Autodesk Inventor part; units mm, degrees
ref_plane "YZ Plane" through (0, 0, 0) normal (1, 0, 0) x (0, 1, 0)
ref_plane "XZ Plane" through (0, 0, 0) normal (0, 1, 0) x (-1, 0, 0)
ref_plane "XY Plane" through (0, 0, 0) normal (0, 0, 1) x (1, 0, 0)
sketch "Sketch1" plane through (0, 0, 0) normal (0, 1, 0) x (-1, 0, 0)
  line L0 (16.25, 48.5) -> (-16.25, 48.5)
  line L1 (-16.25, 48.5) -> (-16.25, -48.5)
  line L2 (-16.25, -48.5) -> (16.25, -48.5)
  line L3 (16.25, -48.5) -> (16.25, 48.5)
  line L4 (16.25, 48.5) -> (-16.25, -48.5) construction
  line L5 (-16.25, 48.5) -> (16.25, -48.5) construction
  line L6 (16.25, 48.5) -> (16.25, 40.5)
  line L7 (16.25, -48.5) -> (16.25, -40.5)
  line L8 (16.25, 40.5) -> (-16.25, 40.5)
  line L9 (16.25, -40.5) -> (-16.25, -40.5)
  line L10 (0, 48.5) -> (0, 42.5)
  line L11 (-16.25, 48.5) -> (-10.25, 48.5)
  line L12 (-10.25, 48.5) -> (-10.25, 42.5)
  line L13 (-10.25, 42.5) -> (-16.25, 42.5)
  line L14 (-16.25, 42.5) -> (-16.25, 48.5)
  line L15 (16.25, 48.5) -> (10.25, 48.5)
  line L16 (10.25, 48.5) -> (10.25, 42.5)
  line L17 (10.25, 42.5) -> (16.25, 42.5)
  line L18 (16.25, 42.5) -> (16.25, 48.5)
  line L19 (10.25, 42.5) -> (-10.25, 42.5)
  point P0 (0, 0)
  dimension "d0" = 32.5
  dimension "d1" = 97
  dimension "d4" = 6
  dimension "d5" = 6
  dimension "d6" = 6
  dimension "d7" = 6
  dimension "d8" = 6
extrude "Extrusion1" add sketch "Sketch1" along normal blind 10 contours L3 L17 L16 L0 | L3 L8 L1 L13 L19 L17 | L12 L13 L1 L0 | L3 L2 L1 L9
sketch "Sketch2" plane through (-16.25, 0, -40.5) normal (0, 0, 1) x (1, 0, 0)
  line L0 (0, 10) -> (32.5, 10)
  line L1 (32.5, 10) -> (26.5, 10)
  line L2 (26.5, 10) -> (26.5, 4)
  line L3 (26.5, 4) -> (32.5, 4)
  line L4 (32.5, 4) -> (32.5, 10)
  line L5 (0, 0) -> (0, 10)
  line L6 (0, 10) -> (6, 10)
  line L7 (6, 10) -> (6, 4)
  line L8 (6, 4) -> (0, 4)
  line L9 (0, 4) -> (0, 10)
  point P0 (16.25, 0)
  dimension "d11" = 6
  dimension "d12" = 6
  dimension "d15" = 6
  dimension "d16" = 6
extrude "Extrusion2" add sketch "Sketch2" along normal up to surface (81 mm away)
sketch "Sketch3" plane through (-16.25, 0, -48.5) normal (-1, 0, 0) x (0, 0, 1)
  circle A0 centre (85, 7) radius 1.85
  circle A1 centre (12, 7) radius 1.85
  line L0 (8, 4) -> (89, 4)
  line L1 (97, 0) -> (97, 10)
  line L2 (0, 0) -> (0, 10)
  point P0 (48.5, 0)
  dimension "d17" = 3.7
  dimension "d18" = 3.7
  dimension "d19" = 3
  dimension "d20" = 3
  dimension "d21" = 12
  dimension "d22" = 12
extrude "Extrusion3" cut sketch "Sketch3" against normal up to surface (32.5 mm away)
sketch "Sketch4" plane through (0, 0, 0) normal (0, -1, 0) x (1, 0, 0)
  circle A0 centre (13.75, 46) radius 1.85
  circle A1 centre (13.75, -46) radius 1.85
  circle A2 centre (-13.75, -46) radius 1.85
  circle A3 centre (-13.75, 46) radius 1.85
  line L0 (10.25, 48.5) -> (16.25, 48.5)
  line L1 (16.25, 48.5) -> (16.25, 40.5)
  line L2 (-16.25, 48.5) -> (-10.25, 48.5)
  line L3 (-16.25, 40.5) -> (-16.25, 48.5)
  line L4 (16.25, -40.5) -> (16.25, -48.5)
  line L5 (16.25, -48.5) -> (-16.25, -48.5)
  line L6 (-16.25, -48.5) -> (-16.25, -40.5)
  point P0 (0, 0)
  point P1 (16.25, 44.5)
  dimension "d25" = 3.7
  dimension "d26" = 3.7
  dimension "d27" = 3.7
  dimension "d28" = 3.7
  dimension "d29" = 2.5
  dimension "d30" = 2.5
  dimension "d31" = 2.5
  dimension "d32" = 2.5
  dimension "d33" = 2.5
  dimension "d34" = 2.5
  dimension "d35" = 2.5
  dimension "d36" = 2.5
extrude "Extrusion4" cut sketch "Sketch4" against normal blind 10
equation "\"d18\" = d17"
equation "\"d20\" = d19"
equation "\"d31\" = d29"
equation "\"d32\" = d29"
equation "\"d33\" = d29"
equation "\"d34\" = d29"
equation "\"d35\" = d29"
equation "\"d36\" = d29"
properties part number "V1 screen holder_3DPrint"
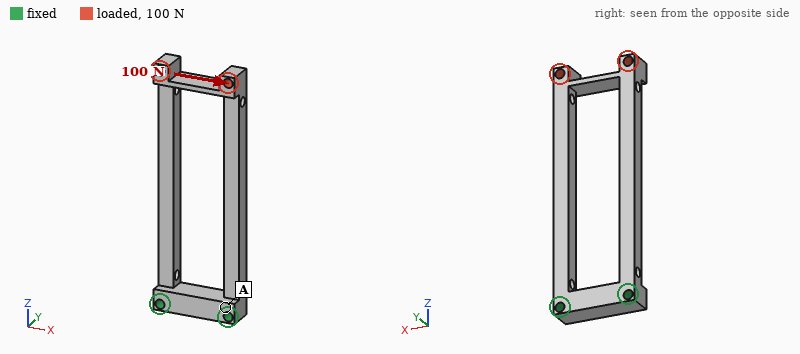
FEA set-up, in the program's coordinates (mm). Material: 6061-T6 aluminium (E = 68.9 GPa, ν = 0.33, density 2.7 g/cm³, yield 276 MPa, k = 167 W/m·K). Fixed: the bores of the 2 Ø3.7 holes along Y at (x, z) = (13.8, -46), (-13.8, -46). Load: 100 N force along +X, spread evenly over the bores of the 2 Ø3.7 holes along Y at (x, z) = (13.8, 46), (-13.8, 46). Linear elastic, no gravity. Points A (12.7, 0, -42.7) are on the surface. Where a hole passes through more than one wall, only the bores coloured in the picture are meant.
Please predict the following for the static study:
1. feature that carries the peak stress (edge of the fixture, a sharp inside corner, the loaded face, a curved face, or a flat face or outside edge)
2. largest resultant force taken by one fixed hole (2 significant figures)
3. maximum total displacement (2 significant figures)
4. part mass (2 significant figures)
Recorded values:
a curved face
240 N
0.93 mm
25 g
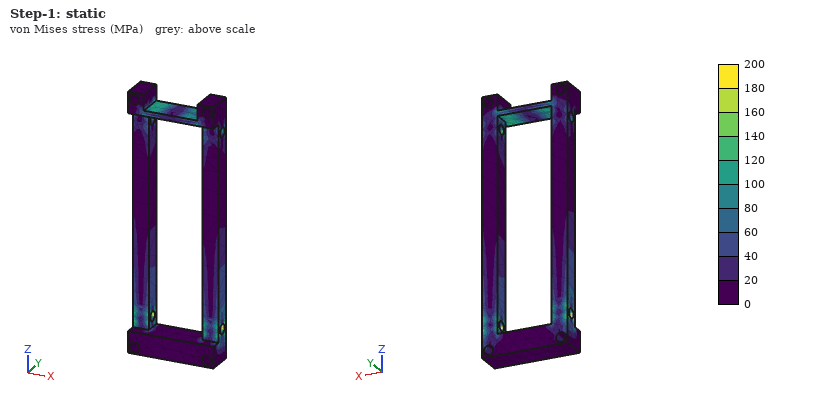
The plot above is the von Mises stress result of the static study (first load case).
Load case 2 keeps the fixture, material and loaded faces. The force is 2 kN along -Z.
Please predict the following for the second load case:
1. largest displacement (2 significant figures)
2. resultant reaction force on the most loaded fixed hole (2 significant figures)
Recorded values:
1.1 mm
1.0 kN
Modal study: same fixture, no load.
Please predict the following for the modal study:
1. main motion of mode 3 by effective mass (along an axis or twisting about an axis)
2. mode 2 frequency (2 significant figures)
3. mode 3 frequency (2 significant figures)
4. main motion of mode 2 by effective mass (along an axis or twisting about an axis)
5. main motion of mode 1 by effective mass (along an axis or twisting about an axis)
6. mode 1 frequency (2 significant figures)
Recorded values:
twisting about Z
630 Hz
1500 Hz
along X
along Y
520 Hz
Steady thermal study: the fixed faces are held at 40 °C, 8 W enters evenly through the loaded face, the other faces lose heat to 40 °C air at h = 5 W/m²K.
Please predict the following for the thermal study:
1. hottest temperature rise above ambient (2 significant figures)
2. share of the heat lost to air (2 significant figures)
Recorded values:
61 K
11 %
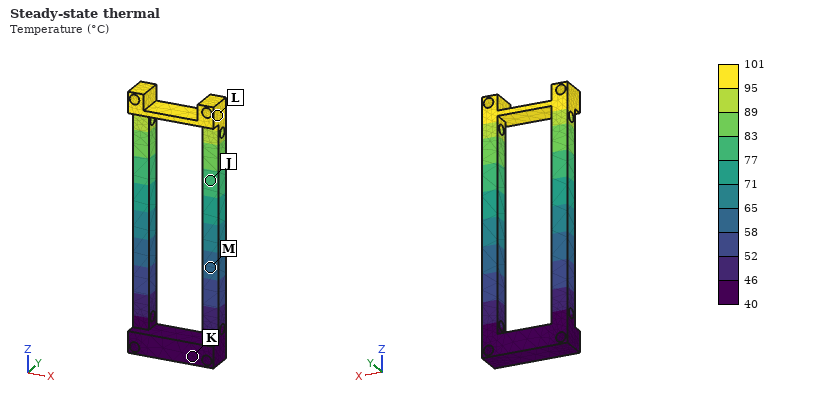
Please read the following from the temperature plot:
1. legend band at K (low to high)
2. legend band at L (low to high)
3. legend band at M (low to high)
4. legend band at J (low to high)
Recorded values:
40 to 46 °C
95 to 101 °C
58 to 65 °C
77 to 83 °C
